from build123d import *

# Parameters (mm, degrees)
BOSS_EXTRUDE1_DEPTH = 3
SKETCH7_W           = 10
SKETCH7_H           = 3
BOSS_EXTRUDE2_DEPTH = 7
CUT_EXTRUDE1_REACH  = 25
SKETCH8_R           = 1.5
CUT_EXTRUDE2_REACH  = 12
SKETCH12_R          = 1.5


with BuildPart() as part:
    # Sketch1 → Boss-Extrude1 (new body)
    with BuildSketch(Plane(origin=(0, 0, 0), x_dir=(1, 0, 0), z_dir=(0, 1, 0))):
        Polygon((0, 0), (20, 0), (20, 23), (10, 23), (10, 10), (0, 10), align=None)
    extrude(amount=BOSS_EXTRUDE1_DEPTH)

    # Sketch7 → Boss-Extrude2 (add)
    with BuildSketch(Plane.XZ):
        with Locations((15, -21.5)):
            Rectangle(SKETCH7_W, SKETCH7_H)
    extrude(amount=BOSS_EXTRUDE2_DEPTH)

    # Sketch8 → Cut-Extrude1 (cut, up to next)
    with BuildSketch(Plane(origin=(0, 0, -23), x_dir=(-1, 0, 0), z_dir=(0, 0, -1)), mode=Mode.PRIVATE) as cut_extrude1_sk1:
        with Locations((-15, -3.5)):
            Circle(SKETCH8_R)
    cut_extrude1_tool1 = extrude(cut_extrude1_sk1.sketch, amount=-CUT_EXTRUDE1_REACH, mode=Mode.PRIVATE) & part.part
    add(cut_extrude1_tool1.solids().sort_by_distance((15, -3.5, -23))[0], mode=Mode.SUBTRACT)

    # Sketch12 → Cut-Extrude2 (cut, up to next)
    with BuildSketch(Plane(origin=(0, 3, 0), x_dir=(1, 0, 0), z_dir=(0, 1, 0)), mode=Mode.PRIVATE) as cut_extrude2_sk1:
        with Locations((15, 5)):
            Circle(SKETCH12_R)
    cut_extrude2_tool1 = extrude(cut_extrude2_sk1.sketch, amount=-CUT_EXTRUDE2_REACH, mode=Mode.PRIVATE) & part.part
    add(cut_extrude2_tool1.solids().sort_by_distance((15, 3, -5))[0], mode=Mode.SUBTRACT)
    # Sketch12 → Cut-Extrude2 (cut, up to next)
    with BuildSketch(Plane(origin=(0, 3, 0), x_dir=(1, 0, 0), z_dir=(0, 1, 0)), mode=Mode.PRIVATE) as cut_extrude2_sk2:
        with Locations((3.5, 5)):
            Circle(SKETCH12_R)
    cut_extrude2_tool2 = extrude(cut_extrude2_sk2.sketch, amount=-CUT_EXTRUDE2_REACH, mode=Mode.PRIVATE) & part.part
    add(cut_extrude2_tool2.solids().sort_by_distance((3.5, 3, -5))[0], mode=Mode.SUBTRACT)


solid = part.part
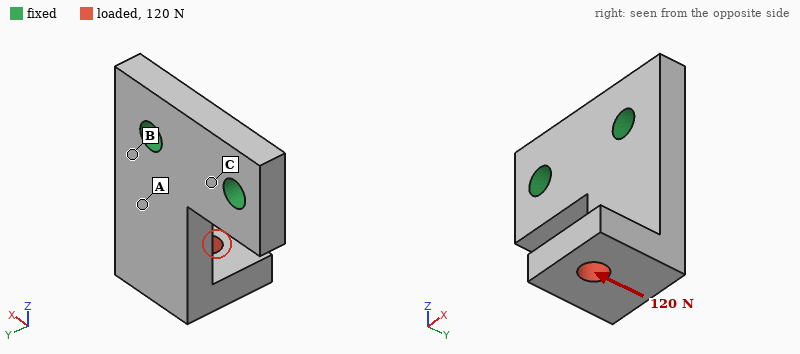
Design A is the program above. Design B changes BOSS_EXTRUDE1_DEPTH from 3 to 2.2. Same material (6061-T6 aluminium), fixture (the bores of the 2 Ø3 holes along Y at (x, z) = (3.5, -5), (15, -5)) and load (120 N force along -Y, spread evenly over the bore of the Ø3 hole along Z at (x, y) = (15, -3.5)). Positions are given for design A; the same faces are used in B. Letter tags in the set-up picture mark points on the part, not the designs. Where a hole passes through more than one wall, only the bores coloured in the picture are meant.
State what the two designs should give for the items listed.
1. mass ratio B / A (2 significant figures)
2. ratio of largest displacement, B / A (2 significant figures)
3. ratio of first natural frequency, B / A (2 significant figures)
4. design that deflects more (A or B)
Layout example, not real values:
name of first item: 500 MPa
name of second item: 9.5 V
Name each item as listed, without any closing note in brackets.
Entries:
mass ratio B / A: 0.78
ratio of largest displacement, B / A: 2.4
ratio of first natural frequency, B / A: 0.69
design that deflects more: B
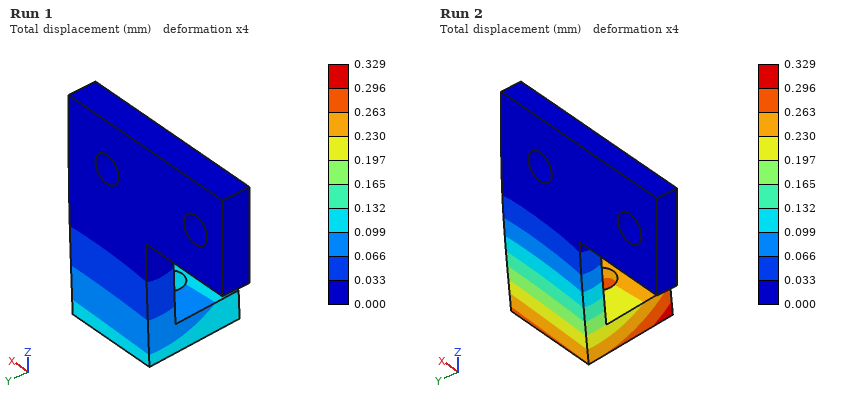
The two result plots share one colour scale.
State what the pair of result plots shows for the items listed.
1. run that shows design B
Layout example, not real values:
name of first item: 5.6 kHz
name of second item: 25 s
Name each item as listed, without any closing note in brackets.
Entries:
run that shows design B: Run 2
